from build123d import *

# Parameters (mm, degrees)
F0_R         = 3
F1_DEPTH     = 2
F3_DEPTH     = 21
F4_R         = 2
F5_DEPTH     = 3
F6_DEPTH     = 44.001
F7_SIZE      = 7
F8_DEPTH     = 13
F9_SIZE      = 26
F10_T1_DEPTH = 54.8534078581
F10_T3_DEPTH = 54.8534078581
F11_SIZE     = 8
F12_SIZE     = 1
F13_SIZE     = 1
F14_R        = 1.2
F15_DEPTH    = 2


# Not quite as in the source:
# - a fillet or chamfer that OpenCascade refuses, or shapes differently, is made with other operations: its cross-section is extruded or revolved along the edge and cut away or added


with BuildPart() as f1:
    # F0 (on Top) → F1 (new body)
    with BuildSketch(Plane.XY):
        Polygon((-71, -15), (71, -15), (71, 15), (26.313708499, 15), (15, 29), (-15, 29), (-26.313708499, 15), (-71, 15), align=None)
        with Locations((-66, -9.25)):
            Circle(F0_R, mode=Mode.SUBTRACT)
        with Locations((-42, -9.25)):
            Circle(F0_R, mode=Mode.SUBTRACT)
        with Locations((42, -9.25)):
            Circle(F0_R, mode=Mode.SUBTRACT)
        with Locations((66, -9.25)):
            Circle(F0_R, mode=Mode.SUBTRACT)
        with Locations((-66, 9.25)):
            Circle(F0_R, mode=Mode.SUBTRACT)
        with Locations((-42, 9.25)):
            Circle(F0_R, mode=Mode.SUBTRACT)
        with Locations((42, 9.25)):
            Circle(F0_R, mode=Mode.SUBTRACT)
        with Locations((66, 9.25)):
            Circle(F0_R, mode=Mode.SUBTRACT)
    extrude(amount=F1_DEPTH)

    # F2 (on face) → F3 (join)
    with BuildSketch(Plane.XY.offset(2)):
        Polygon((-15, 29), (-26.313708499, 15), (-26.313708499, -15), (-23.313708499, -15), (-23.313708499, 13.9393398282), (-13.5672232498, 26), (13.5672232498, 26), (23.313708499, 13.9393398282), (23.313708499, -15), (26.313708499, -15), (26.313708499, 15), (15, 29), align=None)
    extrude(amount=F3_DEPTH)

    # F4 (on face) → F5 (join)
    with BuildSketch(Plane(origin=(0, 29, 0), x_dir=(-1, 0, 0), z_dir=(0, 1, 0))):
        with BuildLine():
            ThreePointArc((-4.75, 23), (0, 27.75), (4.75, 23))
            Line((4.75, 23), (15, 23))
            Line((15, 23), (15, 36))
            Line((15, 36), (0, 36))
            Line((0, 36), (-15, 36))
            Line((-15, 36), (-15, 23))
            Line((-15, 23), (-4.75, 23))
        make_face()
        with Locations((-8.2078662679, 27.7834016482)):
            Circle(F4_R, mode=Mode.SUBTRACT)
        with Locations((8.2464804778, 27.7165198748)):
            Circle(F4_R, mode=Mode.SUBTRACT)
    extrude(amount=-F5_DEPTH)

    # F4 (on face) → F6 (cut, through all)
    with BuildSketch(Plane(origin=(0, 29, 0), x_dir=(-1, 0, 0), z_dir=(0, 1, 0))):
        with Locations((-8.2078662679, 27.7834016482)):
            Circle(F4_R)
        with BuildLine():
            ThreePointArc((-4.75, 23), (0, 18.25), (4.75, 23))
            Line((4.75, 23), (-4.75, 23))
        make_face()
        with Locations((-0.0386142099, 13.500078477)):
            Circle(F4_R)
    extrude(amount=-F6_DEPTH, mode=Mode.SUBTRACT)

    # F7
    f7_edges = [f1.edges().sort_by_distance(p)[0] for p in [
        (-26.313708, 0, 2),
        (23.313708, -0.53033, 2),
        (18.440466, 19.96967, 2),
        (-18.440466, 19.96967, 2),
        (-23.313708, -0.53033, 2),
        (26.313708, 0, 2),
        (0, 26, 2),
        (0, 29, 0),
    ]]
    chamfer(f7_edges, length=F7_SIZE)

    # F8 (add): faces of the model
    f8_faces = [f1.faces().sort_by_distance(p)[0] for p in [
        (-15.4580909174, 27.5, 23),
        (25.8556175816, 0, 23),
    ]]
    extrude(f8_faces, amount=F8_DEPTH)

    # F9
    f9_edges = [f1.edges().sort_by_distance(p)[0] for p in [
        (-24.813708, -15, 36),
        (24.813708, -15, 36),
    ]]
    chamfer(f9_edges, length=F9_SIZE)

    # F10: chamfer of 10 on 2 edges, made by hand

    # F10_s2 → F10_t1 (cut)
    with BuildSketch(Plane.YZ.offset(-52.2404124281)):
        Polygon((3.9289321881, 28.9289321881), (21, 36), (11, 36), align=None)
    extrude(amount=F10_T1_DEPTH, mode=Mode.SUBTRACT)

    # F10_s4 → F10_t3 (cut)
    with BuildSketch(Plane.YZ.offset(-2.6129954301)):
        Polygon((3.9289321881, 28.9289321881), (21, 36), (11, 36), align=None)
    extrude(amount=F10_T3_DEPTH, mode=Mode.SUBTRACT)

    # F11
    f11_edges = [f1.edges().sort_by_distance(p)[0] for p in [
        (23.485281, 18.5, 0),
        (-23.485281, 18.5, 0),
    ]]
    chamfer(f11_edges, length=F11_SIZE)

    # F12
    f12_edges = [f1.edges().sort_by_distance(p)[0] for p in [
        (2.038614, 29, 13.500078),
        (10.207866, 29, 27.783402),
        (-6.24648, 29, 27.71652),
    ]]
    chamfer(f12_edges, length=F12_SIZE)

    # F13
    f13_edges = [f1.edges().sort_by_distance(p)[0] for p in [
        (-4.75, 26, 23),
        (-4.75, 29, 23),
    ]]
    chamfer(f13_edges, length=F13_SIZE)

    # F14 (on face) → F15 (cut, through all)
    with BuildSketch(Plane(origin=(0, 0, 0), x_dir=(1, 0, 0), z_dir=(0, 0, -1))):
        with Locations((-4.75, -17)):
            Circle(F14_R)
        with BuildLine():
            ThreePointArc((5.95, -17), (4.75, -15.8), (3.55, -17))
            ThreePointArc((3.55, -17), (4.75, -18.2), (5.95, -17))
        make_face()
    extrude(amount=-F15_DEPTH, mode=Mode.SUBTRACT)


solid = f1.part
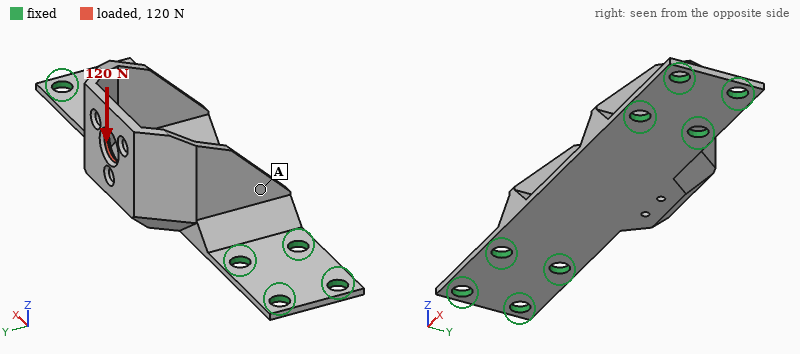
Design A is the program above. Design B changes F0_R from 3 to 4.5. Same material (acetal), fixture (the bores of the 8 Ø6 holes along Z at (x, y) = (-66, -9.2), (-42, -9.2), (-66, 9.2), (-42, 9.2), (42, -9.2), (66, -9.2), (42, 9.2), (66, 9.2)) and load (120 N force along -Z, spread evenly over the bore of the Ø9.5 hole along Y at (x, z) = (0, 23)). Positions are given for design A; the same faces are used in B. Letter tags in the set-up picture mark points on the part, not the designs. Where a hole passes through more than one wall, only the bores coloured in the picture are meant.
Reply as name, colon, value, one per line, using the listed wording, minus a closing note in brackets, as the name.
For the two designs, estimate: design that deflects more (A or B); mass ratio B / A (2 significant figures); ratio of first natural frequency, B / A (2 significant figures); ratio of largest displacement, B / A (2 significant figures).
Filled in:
design that deflects more: A
mass ratio B / A: 0.97
ratio of first natural frequency, B / A: 1.2
ratio of largest displacement, B / A: 0.74
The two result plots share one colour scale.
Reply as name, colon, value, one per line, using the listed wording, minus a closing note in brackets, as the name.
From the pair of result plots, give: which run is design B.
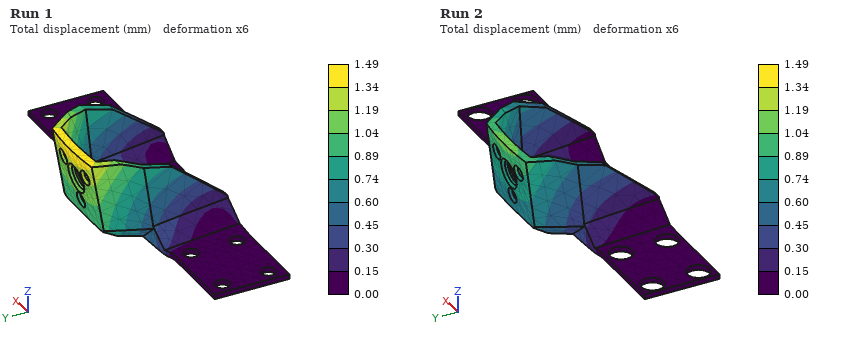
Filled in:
which run is design B: Run 2
